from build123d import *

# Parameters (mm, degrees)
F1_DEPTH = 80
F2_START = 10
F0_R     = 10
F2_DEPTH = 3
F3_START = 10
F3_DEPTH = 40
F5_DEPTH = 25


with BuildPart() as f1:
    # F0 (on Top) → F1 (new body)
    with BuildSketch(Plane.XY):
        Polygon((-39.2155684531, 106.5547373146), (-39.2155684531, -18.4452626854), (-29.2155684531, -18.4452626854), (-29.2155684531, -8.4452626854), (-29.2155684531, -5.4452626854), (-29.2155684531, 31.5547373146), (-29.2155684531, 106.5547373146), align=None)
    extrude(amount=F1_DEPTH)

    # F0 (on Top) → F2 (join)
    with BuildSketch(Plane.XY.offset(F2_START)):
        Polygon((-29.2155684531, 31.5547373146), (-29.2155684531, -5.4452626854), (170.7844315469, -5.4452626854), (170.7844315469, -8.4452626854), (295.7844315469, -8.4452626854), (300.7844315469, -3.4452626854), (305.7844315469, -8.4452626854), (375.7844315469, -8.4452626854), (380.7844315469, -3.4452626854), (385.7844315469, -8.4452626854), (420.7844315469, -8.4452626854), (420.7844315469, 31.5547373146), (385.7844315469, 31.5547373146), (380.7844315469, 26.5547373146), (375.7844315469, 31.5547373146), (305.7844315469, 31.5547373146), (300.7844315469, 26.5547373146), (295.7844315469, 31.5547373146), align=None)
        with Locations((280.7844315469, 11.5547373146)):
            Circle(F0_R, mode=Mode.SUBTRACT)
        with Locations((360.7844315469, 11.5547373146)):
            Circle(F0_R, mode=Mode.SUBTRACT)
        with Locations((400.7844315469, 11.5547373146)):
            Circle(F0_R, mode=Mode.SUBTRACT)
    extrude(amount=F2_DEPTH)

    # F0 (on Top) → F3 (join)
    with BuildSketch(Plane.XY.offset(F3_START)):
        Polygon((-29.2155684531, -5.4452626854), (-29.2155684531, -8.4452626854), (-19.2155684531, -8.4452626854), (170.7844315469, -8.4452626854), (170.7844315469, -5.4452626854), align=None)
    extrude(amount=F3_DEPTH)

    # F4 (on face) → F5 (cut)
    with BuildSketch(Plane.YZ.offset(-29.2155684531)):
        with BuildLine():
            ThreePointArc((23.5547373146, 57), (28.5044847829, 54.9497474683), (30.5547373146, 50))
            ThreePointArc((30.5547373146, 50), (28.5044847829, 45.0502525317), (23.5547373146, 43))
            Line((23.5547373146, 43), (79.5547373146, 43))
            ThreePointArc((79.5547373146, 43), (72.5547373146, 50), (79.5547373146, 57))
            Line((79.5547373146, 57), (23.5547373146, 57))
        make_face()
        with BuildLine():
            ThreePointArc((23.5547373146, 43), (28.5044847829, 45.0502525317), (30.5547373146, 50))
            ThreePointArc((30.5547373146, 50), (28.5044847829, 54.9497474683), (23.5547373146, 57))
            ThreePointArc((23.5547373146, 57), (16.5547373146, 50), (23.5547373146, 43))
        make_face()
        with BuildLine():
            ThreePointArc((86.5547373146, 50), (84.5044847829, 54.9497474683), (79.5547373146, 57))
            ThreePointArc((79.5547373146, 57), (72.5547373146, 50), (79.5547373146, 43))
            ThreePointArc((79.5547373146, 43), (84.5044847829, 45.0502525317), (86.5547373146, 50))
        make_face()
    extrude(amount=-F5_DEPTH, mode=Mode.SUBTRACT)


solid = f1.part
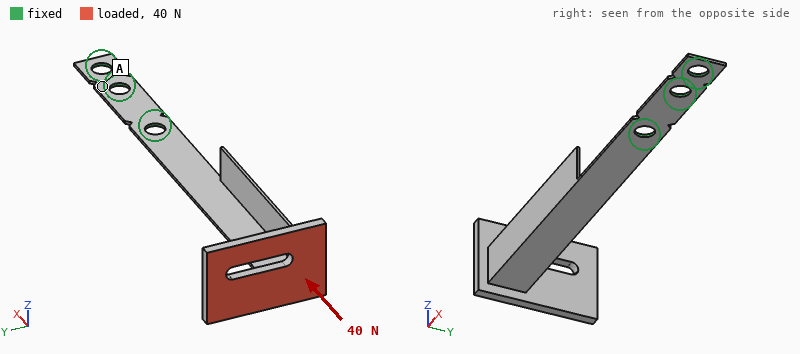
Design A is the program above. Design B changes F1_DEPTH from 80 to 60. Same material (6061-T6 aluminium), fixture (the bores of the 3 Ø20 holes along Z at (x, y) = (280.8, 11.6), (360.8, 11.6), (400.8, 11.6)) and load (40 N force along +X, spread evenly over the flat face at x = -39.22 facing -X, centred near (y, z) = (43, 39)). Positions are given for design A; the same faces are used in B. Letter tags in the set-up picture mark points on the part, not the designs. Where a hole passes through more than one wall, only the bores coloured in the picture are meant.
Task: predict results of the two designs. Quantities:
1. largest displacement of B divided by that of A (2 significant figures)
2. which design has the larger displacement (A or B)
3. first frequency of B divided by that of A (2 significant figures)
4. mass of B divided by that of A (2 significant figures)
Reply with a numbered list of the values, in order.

1. 0.56
2. A
3. 1.1
4. 0.85
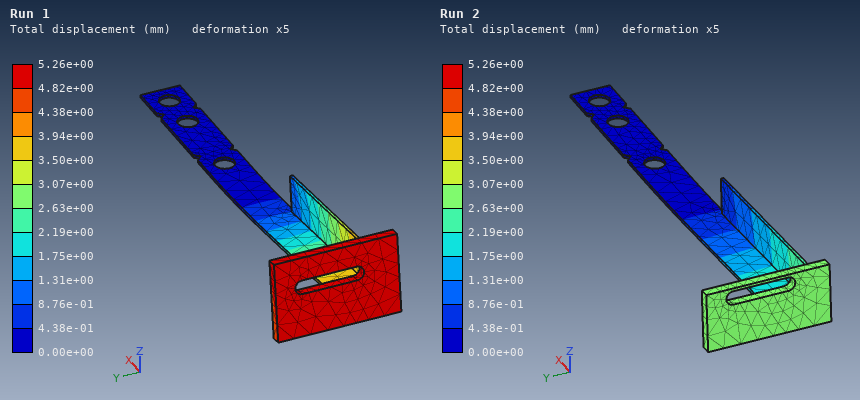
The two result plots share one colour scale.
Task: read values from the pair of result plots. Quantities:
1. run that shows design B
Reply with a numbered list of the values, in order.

1. Run 2
